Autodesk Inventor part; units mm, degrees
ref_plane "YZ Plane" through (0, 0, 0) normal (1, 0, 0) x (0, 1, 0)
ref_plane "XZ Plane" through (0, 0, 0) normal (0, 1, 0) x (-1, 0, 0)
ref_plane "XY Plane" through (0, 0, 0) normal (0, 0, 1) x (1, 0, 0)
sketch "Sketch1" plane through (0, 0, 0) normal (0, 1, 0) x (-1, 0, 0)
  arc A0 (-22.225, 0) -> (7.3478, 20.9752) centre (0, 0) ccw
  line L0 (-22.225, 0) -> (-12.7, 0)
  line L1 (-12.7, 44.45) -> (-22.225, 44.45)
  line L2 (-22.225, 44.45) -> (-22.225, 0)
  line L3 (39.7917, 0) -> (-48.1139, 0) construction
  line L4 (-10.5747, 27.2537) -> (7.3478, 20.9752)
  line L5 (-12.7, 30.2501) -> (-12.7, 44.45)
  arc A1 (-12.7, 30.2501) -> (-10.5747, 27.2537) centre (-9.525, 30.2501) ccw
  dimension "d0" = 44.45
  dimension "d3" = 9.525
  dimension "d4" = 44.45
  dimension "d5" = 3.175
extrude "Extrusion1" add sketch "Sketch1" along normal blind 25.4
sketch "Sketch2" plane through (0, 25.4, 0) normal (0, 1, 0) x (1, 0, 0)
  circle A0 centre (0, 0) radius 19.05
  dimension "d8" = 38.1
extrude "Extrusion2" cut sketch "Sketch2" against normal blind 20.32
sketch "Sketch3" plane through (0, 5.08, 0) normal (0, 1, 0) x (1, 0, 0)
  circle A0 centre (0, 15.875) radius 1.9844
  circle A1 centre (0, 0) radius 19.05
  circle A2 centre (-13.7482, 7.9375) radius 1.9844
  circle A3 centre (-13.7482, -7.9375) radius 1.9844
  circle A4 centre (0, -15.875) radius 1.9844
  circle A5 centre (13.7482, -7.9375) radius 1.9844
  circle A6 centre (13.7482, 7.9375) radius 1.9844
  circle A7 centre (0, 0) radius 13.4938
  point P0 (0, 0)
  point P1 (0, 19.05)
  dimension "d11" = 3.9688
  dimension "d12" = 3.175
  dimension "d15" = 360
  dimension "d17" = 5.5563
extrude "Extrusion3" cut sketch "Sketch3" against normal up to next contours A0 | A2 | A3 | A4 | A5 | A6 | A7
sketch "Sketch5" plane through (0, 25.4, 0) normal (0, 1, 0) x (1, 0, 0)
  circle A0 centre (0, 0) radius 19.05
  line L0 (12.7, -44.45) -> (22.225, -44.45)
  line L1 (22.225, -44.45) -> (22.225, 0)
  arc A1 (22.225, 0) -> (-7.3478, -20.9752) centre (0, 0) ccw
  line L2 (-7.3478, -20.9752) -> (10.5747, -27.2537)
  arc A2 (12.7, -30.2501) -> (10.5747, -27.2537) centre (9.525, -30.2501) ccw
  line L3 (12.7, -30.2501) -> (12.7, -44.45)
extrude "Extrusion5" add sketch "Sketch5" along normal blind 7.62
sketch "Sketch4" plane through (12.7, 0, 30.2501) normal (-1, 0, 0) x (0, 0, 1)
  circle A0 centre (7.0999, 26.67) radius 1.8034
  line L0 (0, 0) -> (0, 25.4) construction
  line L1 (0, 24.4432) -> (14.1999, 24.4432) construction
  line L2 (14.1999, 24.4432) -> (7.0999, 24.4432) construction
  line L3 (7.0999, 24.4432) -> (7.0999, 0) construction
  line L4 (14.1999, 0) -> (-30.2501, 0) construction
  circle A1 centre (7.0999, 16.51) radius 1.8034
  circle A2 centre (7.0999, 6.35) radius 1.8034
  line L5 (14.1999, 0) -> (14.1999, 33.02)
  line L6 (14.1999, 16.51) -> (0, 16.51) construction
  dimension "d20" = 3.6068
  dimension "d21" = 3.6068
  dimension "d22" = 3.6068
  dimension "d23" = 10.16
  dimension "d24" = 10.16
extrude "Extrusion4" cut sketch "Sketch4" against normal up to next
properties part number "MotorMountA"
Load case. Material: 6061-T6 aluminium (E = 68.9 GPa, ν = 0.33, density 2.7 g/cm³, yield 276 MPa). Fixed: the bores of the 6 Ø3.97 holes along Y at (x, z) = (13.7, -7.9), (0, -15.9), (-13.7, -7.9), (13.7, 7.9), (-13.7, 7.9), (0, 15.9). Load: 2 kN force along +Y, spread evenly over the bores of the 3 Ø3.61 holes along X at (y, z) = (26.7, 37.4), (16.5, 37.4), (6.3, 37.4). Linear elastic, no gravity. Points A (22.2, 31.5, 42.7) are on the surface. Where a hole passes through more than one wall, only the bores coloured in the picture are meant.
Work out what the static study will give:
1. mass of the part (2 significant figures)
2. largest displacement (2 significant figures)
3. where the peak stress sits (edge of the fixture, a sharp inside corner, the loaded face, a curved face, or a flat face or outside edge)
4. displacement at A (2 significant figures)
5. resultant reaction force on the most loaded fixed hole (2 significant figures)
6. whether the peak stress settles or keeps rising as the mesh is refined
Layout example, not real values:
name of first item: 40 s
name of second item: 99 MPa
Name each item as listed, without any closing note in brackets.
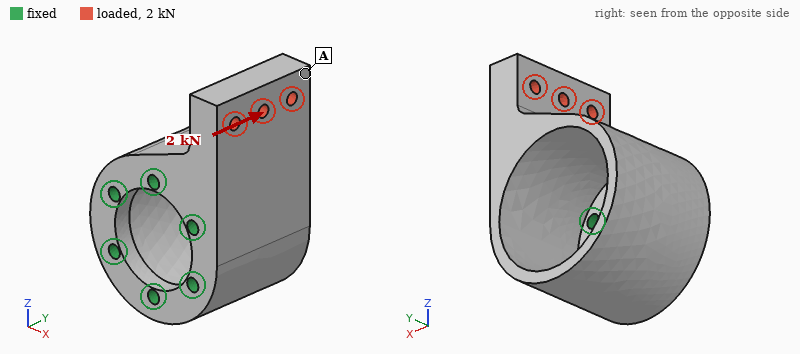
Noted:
mass of the part: 75 g
largest displacement: 99 µm
where the peak stress sits: edge of the fixture
displacement at A: 94 µm
resultant reaction force on the most loaded fixed hole: 2.1 kN
whether the peak stress settles or keeps rising as the mesh is refined: keeps rising
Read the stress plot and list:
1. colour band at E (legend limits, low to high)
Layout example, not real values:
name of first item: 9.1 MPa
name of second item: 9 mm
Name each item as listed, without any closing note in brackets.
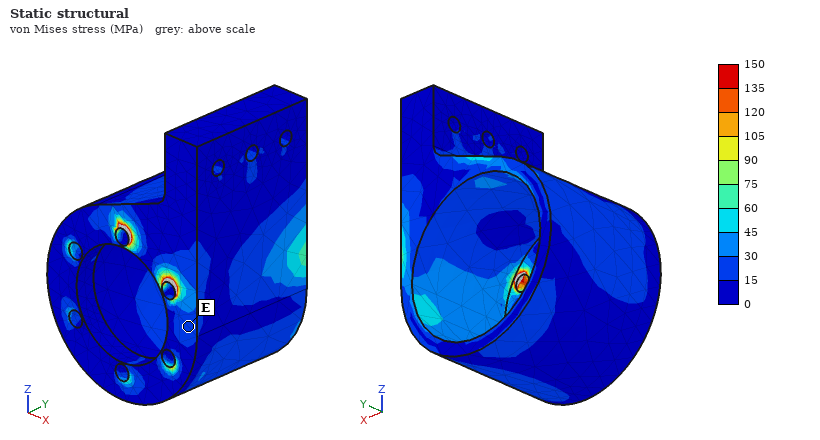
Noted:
colour band at E: 15 to 30 MPa
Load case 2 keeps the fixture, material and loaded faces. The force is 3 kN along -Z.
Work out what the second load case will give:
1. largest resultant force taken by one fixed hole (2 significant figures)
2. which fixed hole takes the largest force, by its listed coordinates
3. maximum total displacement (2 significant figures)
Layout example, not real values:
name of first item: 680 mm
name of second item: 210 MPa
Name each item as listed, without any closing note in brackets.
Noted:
largest resultant force taken by one fixed hole: 1.9 kN
which fixed hole takes the largest force, by its listed coordinates: (13.7, 7.9)
maximum total displacement: 58 µm
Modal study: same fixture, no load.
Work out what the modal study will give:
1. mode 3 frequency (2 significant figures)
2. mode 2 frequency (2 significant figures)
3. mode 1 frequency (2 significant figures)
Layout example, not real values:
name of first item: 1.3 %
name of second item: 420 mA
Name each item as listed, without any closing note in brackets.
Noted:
mode 3 frequency: 9000 Hz
mode 2 frequency: 8600 Hz
mode 1 frequency: 5100 Hz
